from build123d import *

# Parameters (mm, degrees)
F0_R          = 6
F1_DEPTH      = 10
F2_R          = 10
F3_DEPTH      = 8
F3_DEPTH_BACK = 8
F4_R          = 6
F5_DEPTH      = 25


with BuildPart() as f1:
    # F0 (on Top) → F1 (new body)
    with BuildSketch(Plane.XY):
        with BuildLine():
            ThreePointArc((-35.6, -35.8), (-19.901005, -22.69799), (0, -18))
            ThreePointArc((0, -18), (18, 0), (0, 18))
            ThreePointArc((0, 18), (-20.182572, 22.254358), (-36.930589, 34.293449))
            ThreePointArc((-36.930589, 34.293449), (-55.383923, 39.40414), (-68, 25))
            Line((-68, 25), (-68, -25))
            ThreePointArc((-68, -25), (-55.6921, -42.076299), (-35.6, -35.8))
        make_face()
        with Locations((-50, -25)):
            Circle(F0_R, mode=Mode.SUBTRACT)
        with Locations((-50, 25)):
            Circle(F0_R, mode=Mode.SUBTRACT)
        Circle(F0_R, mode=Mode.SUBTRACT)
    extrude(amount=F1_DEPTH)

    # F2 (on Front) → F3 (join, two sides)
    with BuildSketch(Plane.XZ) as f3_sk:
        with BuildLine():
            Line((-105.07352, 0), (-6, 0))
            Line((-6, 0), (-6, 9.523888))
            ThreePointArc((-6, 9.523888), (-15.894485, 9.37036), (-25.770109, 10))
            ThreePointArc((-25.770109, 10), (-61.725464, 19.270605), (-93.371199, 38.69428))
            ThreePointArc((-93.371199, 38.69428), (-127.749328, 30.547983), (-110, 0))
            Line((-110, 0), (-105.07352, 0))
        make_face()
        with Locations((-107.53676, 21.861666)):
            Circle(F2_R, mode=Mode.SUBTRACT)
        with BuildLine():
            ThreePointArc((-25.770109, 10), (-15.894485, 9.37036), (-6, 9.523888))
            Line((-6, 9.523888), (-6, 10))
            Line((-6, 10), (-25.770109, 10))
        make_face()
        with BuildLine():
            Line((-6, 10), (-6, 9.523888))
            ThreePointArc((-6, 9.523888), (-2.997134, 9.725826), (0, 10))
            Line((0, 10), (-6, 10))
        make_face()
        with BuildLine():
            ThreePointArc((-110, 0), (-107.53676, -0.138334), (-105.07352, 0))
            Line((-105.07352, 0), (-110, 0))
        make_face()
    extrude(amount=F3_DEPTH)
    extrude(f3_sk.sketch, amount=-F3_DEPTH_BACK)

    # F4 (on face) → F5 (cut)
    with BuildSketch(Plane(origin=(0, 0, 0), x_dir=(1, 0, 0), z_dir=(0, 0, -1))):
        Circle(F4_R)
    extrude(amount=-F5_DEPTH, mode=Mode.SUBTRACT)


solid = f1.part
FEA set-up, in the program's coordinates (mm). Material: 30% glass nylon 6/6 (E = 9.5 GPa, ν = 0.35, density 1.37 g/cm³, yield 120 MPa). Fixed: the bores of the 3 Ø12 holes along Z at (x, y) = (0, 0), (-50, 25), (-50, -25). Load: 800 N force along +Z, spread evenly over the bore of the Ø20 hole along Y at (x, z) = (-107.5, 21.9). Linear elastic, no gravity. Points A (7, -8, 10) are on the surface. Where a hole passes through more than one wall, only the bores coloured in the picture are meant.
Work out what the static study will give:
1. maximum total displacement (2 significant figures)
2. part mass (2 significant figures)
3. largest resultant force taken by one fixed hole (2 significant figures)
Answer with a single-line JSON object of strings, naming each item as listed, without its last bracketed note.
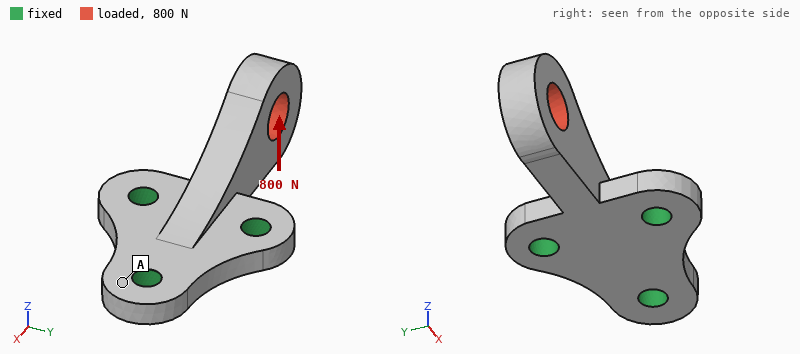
{"maximum total displacement": "1.1 mm", "part mass": "100 g", "largest resultant force taken by one fixed hole": "770 N"}
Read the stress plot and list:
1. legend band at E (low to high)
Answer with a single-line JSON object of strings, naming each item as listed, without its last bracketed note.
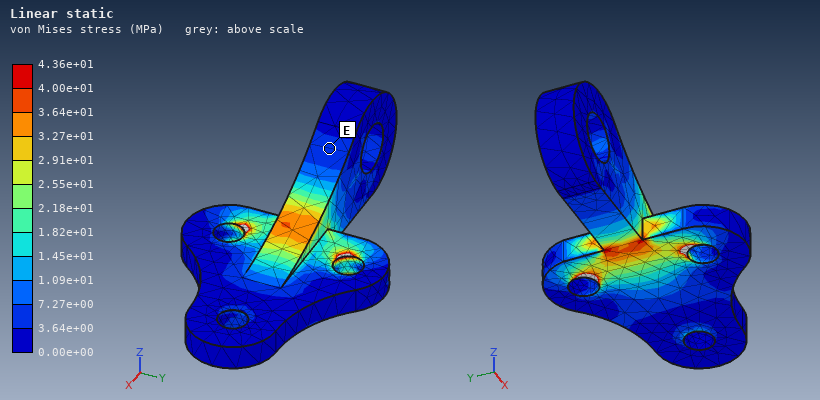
{"legend band at E": "3.64e+00 to 7.27e+00 MPa"}
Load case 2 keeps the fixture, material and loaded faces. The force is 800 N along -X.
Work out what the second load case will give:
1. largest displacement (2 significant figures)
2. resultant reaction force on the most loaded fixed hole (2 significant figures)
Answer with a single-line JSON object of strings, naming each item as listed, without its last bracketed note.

{"largest displacement": "0.33 mm", "resultant reaction force on the most loaded fixed hole": "280 N"}
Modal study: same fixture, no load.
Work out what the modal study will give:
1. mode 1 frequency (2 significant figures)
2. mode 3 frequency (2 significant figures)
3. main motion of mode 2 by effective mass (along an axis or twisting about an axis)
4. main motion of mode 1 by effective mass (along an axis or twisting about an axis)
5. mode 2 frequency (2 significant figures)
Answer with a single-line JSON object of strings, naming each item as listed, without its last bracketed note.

{"mode 1 frequency": "870 Hz", "mode 3 frequency": "2800 Hz", "main motion of mode 2 by effective mass": "along Y", "main motion of mode 1 by effective mass": "along Z", "mode 2 frequency": "1100 Hz"}
